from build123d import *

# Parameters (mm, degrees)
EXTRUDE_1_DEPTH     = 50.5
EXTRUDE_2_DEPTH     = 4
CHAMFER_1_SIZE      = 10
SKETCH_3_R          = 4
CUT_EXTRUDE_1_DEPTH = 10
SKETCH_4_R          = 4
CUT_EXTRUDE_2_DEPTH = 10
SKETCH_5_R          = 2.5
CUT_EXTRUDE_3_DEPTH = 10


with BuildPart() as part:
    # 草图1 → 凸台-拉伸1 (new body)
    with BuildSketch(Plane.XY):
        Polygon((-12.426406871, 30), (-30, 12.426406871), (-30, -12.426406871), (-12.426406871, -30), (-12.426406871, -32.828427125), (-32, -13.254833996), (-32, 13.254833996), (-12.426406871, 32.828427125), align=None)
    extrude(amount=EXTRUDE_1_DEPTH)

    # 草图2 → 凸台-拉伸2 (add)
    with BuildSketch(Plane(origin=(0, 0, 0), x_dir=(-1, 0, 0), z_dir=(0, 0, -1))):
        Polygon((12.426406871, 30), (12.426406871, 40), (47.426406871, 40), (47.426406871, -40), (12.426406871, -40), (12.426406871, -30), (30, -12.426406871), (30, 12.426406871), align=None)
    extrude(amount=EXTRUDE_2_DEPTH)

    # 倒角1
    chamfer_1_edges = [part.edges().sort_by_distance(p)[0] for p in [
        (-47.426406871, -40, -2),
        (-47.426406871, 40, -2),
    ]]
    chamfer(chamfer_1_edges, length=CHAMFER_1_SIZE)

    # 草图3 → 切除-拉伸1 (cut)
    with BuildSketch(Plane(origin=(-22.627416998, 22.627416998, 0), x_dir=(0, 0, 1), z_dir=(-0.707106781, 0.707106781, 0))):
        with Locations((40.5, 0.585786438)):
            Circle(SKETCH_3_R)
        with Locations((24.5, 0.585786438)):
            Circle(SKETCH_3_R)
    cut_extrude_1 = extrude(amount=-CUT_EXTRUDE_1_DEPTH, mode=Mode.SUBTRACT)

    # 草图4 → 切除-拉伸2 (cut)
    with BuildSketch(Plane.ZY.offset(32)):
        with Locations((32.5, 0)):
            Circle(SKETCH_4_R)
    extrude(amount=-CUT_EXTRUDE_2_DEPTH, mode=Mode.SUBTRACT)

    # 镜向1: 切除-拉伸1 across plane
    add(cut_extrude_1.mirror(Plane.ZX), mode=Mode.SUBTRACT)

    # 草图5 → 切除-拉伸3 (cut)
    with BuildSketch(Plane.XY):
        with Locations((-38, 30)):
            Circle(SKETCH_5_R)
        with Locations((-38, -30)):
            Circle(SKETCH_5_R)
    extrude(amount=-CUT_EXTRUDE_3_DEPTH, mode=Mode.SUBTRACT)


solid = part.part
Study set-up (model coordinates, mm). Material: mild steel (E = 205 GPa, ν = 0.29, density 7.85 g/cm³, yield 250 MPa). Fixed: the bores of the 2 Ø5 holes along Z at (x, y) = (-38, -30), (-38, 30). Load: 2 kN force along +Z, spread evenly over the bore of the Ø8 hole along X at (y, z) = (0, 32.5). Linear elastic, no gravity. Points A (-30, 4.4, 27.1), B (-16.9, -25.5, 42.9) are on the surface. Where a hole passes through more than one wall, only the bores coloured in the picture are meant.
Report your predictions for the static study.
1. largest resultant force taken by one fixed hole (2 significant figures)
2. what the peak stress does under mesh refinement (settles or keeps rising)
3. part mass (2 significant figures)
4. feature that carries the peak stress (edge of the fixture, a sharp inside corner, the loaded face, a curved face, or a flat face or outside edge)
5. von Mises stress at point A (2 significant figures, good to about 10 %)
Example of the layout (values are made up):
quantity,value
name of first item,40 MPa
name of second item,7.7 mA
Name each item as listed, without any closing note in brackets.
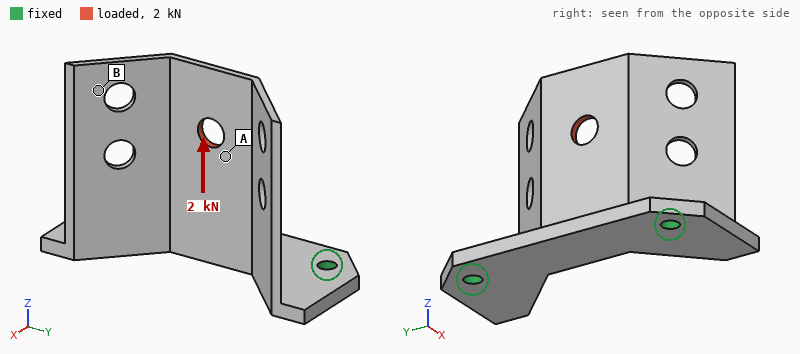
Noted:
quantity,value
largest resultant force taken by one fixed hole,1.1 kN
what the peak stress does under mesh refinement,keeps rising
part mass,120 g
feature that carries the peak stress,edge of the fixture
von Mises stress at point A,43 MPa
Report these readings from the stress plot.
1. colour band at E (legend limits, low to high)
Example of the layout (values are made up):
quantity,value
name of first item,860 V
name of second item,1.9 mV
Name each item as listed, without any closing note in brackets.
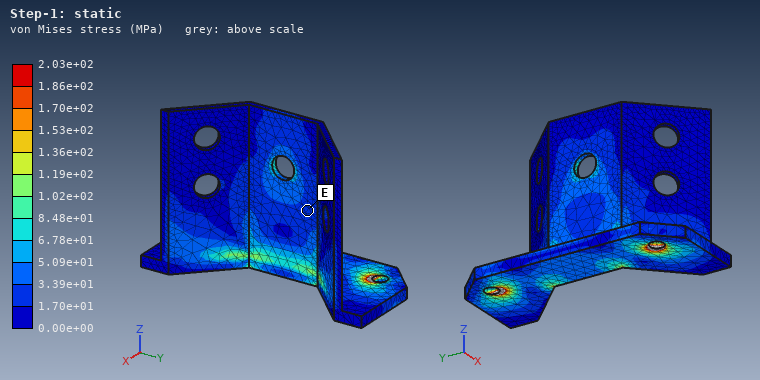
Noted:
quantity,value
colour band at E,1.70e+01 to 3.39e+01 MPa
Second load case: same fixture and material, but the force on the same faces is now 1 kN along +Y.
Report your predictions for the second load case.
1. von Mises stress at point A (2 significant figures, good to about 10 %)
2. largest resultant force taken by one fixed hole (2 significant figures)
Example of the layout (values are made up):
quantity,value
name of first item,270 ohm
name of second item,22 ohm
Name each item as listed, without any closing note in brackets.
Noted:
quantity,value
von Mises stress at point A,43 MPa
largest resultant force taken by one fixed hole,880 N
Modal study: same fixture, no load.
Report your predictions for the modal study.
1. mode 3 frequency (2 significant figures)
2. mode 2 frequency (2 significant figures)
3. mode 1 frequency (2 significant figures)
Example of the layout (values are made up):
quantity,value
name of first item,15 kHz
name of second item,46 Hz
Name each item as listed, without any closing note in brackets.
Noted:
quantity,value
mode 3 frequency,2300 Hz
mode 2 frequency,1300 Hz
mode 1 frequency,1300 Hz
